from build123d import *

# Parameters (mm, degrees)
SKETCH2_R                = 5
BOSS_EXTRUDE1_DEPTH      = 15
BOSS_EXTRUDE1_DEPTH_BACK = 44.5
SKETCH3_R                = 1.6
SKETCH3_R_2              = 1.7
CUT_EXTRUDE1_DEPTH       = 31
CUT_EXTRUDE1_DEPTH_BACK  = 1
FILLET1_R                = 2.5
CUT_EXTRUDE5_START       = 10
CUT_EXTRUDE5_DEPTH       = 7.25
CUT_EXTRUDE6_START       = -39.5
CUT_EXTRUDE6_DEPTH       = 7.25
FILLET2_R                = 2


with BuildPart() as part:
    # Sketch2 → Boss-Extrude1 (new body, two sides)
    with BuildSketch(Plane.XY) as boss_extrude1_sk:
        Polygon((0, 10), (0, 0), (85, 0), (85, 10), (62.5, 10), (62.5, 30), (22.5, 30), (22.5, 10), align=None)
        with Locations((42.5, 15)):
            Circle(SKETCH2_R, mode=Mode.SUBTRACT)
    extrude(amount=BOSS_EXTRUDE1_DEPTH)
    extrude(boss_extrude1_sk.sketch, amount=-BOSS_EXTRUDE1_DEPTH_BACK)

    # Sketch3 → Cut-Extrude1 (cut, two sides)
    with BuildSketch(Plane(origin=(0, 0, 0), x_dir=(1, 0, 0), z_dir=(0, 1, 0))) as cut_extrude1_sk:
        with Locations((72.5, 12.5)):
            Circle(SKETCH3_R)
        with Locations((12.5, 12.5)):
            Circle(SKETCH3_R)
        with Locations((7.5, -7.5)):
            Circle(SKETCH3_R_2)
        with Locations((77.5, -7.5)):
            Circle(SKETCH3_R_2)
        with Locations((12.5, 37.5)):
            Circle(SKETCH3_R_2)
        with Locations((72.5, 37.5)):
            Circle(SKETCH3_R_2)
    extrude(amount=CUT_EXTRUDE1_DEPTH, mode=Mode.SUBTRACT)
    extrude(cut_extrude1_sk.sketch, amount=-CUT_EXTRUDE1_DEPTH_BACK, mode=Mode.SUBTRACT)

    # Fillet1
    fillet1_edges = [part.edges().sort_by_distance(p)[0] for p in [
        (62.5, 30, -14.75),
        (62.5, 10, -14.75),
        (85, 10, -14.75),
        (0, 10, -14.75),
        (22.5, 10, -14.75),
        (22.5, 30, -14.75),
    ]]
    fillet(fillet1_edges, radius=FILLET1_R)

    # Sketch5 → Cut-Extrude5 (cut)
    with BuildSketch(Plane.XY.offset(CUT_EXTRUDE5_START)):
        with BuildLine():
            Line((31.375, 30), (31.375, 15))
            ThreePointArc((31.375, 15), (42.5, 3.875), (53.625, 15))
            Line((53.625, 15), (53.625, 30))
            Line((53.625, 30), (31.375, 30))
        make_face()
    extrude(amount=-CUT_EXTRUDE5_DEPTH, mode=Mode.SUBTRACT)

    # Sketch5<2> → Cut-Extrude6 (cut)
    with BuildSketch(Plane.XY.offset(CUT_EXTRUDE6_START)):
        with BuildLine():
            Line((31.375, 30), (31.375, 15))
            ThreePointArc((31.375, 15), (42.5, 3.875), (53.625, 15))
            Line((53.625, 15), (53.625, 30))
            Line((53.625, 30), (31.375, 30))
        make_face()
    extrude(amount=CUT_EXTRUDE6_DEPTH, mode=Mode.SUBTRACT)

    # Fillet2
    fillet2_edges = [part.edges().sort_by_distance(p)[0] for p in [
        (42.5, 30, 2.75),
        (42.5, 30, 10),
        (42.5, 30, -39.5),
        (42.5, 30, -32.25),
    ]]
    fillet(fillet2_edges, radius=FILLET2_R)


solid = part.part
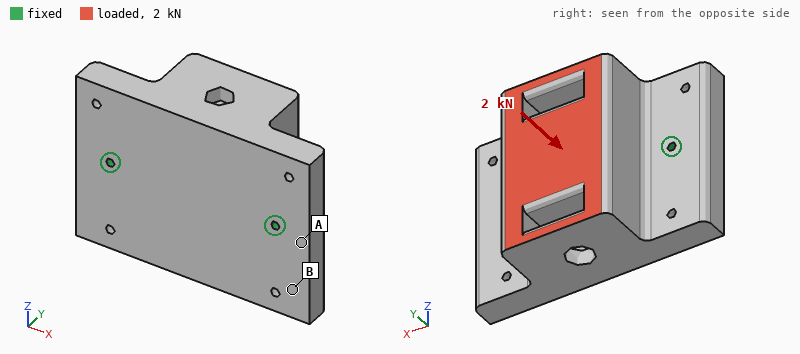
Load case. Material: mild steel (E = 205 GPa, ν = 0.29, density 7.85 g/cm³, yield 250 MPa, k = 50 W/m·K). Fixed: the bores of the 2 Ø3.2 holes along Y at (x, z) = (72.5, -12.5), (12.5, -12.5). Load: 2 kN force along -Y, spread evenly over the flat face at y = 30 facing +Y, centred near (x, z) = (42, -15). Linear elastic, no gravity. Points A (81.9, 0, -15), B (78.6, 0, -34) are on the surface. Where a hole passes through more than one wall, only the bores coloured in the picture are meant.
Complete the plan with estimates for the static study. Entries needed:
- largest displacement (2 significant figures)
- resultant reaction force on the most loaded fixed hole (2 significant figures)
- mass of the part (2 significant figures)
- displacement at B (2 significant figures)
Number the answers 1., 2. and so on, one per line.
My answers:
1. 3.8 µm
2. 1.1 kN
3. 680 g
4. 1.7 µm
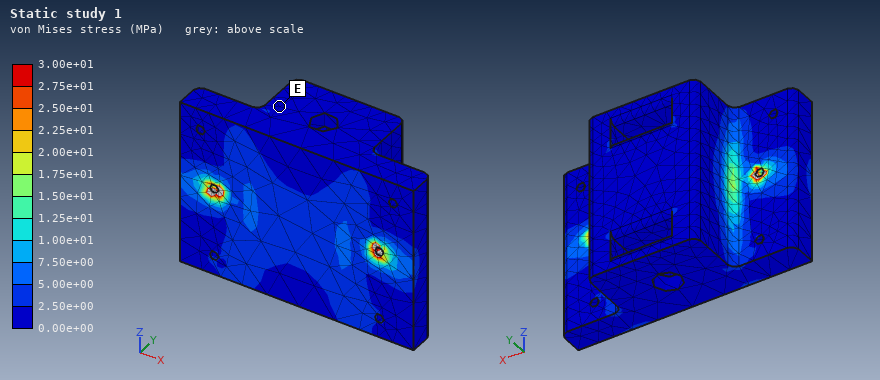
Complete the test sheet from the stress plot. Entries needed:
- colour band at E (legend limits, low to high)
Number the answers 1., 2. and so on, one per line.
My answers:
1. 0.00e+00 to 2.50e+00 MPa
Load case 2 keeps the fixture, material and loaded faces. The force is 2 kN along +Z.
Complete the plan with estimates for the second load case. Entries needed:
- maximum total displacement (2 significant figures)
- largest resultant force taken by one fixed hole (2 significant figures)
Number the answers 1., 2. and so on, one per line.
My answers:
1. 23 µm
2. 1.0 kN
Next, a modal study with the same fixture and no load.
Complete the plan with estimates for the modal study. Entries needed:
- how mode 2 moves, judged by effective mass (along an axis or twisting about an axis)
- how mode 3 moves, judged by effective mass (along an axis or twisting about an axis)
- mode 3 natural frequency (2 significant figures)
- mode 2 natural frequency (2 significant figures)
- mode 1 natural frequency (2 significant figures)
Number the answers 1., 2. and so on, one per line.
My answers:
1. along Y
2. along X
3. 9800 Hz
4. 7300 Hz
5. 3000 Hz
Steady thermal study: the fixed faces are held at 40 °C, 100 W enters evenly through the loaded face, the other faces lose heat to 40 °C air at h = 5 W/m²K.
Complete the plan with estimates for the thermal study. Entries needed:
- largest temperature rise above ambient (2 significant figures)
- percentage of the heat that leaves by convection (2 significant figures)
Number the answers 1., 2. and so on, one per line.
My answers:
1. 78 K
2. 4.6 %
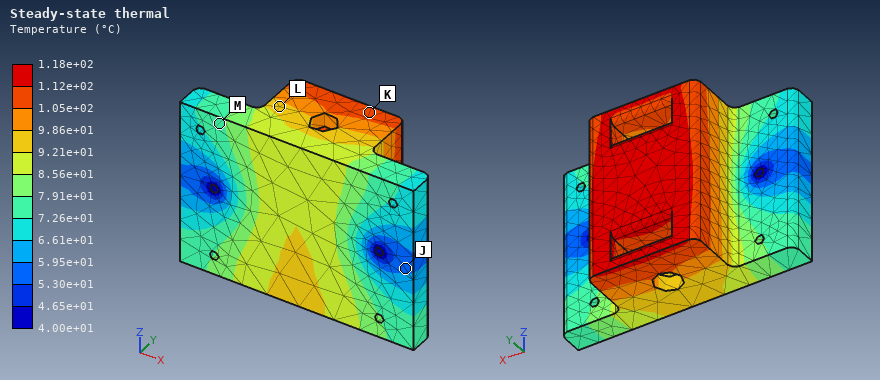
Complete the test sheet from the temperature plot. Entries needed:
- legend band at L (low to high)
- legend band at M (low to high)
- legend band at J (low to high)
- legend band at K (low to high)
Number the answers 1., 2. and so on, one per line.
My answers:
1. 9.21e+01 to 9.86e+01 °C
2. 7.26e+01 to 7.91e+01 °C
3. 5.30e+01 to 5.95e+01 °C
4. 1.05e+02 to 1.12e+02 °C
